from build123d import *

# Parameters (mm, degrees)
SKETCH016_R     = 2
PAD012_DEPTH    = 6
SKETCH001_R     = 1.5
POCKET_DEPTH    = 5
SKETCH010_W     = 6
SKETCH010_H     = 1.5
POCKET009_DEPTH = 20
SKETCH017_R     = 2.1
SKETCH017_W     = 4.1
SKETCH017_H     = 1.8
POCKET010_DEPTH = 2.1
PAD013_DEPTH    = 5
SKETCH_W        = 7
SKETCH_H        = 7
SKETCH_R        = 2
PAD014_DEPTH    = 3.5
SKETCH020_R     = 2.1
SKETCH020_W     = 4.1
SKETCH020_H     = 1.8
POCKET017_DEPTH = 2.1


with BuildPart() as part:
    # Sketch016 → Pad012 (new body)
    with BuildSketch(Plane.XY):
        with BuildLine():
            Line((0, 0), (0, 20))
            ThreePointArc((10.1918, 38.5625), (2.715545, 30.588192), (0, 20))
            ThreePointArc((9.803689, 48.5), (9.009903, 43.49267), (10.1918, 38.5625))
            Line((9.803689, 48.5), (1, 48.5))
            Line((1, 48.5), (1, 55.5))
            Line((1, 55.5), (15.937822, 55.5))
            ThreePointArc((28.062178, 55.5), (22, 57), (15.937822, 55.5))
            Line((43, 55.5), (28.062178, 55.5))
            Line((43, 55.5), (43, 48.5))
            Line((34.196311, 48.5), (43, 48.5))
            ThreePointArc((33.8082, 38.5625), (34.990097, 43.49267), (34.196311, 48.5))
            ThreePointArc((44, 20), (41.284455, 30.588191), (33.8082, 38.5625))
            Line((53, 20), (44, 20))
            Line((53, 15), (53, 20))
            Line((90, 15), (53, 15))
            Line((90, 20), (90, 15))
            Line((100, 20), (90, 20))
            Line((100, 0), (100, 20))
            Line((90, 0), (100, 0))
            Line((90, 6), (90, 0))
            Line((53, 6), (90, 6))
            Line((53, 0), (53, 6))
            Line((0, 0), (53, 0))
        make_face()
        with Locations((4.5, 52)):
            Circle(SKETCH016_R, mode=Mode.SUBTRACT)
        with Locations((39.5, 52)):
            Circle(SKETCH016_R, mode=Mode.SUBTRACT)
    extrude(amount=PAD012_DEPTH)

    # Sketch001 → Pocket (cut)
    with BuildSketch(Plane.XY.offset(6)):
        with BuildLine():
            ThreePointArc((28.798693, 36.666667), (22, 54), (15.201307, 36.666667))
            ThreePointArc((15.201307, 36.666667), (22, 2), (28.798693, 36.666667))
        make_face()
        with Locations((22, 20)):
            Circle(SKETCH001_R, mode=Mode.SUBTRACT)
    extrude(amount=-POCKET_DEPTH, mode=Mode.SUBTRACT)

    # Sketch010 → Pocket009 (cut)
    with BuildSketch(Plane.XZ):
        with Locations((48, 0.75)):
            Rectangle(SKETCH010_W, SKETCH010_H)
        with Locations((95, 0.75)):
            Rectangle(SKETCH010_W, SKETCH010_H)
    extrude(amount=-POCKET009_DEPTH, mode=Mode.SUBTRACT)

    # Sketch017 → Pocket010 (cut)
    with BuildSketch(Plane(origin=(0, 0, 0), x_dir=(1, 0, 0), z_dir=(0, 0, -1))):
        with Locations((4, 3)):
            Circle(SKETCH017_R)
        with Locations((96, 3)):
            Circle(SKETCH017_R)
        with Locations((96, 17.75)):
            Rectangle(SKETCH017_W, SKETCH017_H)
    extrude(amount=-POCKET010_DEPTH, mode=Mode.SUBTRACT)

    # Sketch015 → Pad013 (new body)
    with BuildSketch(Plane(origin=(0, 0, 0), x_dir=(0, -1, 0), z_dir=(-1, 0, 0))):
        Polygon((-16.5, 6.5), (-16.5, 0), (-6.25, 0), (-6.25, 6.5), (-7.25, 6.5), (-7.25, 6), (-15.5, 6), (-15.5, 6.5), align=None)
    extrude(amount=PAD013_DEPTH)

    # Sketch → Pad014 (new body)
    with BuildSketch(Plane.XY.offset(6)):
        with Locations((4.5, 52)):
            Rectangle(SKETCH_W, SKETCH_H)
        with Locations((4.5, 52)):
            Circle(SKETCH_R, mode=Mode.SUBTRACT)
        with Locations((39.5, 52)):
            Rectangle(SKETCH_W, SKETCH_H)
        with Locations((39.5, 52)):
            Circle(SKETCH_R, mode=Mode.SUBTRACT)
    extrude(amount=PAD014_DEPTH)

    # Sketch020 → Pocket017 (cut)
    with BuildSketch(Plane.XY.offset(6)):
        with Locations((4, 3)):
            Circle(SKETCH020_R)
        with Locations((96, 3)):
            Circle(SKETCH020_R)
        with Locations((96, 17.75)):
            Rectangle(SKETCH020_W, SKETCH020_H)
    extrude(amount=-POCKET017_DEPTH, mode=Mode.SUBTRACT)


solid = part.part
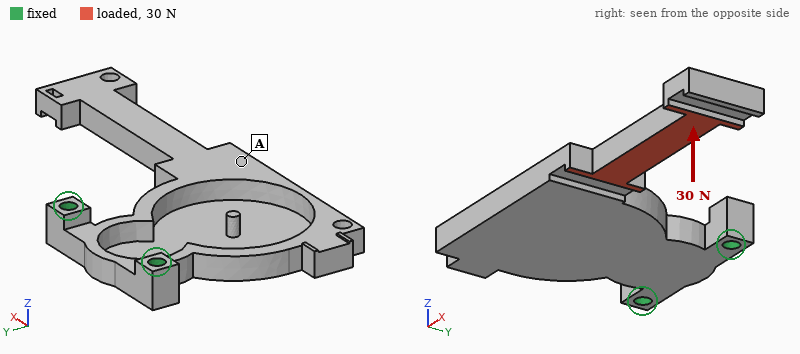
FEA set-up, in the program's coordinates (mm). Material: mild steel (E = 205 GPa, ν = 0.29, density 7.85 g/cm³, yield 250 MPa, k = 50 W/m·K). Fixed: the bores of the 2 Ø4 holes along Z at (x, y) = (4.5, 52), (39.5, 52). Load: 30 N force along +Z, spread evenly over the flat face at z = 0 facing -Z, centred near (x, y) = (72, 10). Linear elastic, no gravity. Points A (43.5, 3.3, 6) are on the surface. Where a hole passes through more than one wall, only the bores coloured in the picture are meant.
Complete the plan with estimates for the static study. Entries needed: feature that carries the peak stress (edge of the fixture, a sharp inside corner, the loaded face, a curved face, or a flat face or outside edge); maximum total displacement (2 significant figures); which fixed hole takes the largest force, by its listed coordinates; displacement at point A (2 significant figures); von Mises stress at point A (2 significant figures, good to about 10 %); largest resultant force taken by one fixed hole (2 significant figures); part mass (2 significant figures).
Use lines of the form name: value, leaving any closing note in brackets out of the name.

feature that carries the peak stress: a curved face
maximum total displacement: 0.24 mm
which fixed hole takes the largest force, by its listed coordinates: (39.5, 52)
displacement at point A: 0.080 mm
von Mises stress at point A: 9.0 MPa
largest resultant force taken by one fixed hole: 74 N
part mass: 84 g
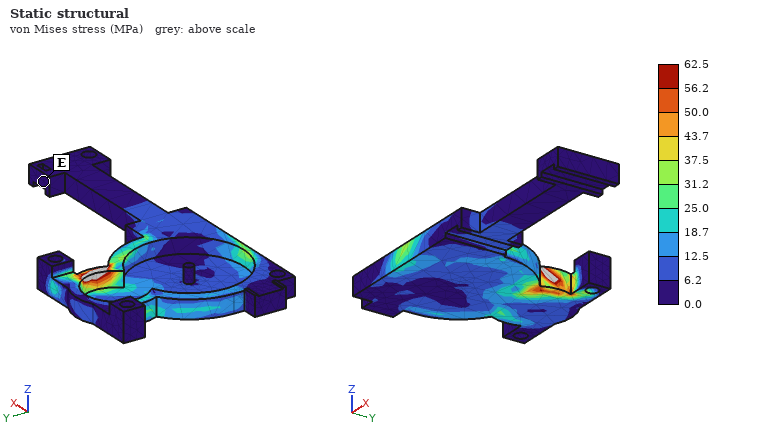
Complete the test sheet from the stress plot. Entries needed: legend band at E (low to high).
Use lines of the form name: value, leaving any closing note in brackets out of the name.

legend band at E: 0.0 to 6.2 MPa
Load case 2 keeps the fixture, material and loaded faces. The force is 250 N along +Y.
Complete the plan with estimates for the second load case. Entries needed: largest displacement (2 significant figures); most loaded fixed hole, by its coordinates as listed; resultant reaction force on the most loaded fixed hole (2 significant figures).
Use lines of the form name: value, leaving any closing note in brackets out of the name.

largest displacement: 0.19 mm
most loaded fixed hole, by its coordinates as listed: (39.5, 52)
resultant reaction force on the most loaded fixed hole: 590 N
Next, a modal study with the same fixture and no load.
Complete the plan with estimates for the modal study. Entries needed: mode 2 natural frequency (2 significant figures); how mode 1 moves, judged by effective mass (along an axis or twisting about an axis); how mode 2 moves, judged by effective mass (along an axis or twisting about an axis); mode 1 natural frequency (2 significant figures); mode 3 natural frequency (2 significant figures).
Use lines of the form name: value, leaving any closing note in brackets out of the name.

mode 2 natural frequency: 890 Hz
how mode 1 moves, judged by effective mass: along Z
how mode 2 moves, judged by effective mass: along Z
mode 1 natural frequency: 370 Hz
mode 3 natural frequency: 1500 Hz
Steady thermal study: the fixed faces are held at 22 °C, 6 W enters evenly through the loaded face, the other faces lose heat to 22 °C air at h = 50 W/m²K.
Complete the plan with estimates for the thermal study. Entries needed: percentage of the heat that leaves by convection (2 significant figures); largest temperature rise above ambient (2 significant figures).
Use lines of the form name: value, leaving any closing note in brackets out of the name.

percentage of the heat that leaves by convection: 89 %
largest temperature rise above ambient: 40 K
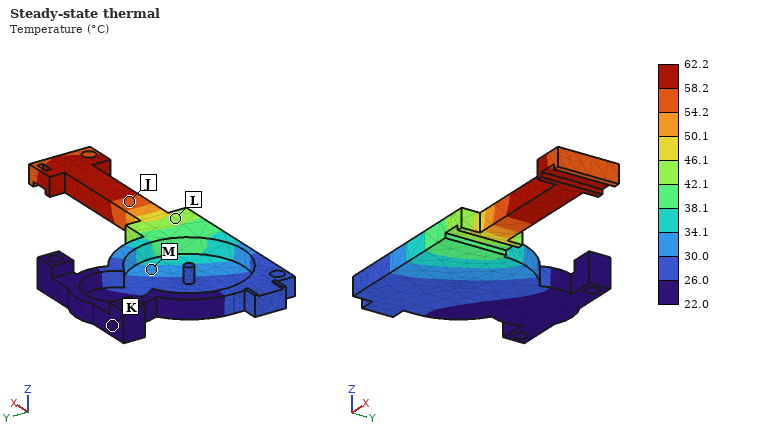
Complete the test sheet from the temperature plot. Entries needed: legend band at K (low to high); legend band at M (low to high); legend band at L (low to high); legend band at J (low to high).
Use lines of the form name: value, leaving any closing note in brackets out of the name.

legend band at K: 22.0 to 26.0 °C
legend band at M: 30.0 to 34.1 °C
legend band at L: 42.1 to 46.1 °C
legend band at J: 54.2 to 58.2 °C
